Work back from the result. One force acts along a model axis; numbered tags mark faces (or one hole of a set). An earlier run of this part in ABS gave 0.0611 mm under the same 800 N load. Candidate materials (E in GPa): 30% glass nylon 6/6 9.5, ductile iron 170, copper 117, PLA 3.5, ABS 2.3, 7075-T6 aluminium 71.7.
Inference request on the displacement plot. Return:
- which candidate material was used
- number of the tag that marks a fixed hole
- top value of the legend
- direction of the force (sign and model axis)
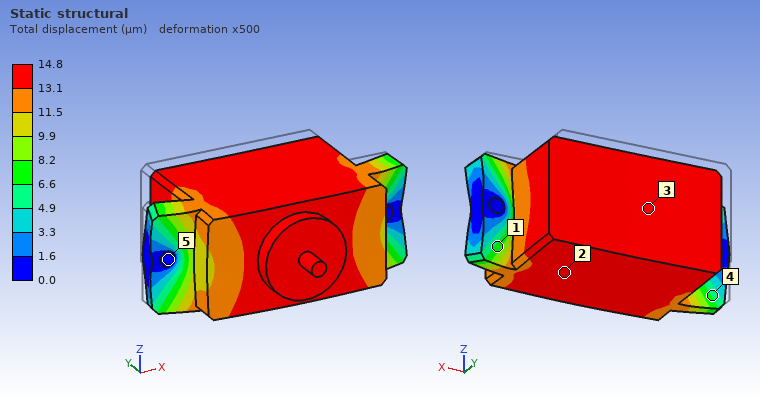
30% glass nylon 6/6
5
14.8 µm
-Y
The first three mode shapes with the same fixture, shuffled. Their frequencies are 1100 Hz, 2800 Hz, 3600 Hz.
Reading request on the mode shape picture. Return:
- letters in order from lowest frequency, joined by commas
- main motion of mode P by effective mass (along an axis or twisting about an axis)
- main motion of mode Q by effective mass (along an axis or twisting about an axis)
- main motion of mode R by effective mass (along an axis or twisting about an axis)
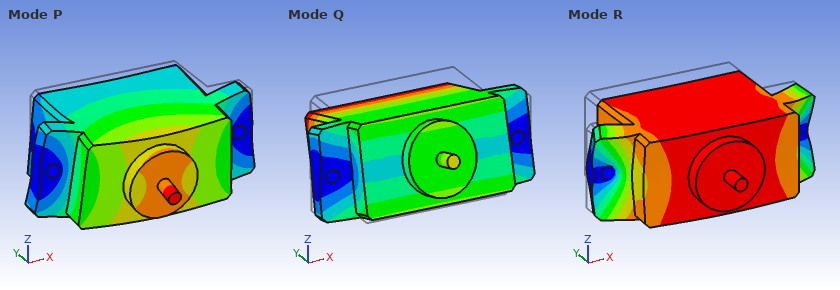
Q, R, P
along Z
along Z
along Y
